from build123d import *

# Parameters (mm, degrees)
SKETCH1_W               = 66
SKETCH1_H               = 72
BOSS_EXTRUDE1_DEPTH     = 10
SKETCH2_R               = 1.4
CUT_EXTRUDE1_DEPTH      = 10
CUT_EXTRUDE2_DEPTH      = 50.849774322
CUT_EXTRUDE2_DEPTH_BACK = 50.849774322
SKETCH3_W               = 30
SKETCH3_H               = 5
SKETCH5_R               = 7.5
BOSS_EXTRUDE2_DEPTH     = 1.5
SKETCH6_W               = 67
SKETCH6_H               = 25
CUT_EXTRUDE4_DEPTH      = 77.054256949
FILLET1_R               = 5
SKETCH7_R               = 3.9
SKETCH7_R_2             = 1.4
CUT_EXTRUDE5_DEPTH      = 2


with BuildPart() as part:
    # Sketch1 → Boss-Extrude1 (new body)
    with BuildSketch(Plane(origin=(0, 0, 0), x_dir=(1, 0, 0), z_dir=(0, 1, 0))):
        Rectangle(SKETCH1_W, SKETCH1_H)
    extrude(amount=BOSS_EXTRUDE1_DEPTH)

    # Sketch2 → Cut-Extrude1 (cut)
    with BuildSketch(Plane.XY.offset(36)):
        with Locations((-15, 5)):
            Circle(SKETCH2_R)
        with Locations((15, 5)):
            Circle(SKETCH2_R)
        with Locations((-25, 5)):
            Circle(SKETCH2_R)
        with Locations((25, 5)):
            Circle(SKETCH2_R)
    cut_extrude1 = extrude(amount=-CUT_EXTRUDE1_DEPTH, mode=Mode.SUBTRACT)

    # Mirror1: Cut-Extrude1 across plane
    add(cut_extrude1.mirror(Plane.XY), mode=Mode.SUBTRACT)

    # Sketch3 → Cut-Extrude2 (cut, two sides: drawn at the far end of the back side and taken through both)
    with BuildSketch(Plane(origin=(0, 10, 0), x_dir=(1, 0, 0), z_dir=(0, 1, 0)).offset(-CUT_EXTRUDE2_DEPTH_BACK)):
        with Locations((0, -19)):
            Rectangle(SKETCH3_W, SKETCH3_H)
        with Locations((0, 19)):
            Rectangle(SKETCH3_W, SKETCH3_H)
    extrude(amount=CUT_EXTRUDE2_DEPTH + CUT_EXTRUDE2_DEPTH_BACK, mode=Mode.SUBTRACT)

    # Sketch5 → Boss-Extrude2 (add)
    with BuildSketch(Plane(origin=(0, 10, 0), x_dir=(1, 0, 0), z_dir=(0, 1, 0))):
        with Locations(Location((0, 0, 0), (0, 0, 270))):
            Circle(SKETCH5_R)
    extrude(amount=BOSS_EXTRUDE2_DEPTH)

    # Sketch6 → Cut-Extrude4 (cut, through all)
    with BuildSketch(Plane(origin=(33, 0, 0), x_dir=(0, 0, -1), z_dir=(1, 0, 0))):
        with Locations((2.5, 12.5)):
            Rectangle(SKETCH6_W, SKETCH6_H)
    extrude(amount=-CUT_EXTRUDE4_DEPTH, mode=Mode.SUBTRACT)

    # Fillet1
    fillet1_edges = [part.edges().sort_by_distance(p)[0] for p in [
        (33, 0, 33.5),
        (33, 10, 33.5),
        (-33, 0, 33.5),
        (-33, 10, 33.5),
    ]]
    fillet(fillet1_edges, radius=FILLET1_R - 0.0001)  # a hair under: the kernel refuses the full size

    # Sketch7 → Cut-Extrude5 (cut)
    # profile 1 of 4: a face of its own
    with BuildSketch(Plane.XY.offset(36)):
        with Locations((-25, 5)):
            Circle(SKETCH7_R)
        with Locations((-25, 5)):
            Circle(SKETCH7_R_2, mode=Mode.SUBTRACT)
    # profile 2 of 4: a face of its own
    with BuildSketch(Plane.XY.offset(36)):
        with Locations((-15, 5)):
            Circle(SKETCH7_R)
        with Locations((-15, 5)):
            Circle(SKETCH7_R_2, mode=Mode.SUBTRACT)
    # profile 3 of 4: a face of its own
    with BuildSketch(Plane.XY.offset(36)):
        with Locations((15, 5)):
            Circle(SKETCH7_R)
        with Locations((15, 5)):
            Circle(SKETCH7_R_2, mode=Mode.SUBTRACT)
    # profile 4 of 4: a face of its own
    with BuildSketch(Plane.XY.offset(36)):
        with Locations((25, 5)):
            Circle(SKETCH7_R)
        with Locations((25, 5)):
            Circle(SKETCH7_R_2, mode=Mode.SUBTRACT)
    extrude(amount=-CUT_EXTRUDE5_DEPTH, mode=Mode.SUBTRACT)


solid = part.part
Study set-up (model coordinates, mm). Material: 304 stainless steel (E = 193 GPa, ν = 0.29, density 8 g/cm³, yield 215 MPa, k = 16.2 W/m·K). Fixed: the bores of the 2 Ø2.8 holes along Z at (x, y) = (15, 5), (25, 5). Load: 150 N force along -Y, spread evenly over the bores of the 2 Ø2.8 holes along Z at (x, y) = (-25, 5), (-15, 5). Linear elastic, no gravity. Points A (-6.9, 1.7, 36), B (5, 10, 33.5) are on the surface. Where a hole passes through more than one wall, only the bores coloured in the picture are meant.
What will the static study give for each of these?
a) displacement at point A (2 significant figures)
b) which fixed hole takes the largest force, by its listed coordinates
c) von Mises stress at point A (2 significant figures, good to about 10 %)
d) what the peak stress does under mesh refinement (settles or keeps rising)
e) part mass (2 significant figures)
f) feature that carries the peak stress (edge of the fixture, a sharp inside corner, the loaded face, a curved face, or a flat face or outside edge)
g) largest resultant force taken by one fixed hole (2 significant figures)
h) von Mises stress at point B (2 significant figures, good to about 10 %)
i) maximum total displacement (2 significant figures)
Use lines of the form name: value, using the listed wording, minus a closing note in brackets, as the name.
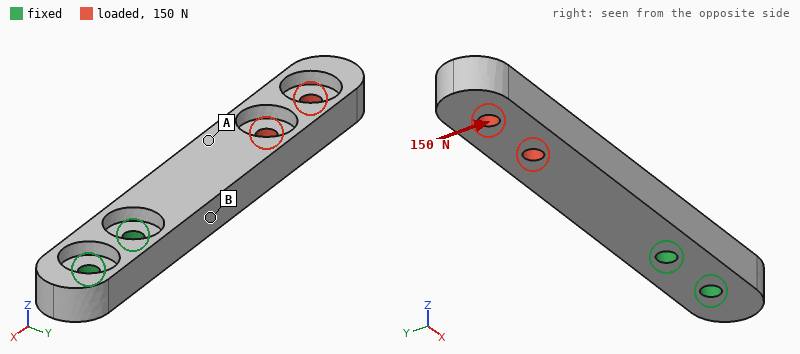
displacement at point A: 21 µm
which fixed hole takes the largest force, by its listed coordinates: (15, 5)
von Mises stress at point A: 14 MPa
what the peak stress does under mesh refinement: keeps rising
part mass: 22 g
feature that carries the peak stress: edge of the fixture
largest resultant force taken by one fixed hole: 470 N
von Mises stress at point B: 45 MPa
maximum total displacement: 62 µm
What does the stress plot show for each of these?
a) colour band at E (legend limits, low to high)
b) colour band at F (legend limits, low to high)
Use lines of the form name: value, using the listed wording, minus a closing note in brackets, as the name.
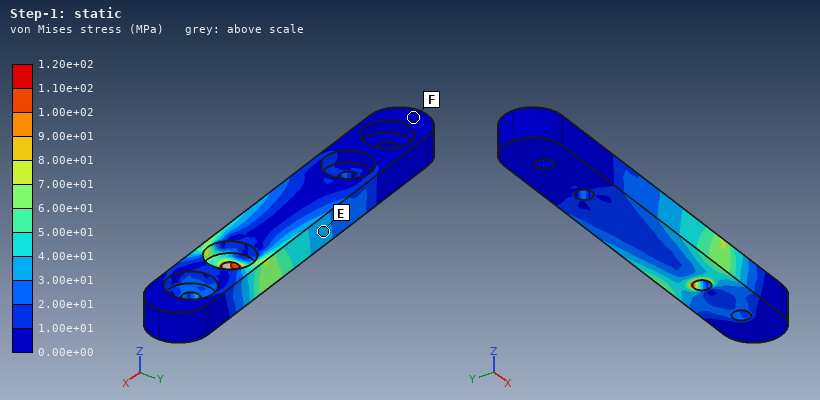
colour band at E: 3.00e+01 to 4.00e+01 MPa
colour band at F: 0.00e+00 to 1.00e+01 MPa
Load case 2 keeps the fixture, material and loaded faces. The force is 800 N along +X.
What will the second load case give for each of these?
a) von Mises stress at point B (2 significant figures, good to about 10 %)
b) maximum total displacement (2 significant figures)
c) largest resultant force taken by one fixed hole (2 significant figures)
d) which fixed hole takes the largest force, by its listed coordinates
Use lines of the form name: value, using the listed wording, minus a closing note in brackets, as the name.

von Mises stress at point B: 16 MPa
maximum total displacement: 38 µm
largest resultant force taken by one fixed hole: 690 N
which fixed hole takes the largest force, by its listed coordinates: (15, 5)
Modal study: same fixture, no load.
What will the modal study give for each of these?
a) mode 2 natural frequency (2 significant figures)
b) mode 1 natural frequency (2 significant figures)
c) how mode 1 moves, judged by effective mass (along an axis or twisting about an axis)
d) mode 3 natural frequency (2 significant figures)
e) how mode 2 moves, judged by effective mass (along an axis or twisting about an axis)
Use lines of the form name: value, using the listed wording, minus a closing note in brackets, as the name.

mode 2 natural frequency: 3200 Hz
mode 1 natural frequency: 1600 Hz
how mode 1 moves, judged by effective mass: along Z
mode 3 natural frequency: 8700 Hz
how mode 2 moves, judged by effective mass: along Y
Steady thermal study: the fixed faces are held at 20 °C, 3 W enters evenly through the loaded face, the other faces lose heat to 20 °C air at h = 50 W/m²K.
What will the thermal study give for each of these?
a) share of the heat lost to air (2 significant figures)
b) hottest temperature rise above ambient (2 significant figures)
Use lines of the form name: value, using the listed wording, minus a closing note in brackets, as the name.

share of the heat lost to air: 76 %
hottest temperature rise above ambient: 54 K
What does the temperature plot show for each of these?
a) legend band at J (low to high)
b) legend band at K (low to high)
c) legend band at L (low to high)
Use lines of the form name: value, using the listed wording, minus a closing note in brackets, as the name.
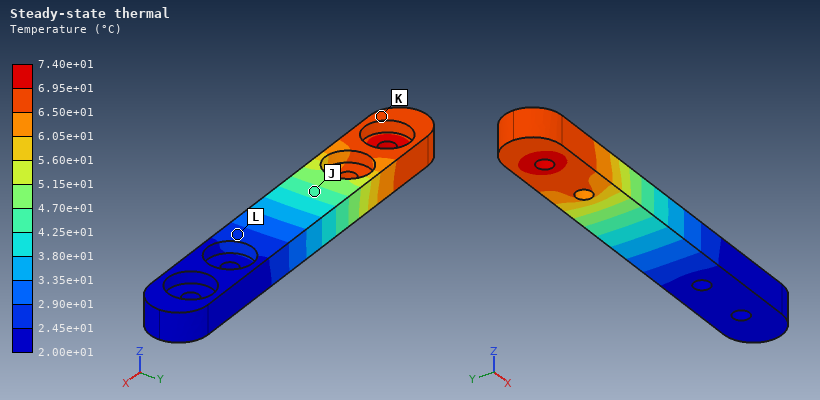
legend band at J: 4.25e+01 to 4.70e+01 °C
legend band at K: 6.50e+01 to 6.95e+01 °C
legend band at L: 2.45e+01 to 2.90e+01 °C
